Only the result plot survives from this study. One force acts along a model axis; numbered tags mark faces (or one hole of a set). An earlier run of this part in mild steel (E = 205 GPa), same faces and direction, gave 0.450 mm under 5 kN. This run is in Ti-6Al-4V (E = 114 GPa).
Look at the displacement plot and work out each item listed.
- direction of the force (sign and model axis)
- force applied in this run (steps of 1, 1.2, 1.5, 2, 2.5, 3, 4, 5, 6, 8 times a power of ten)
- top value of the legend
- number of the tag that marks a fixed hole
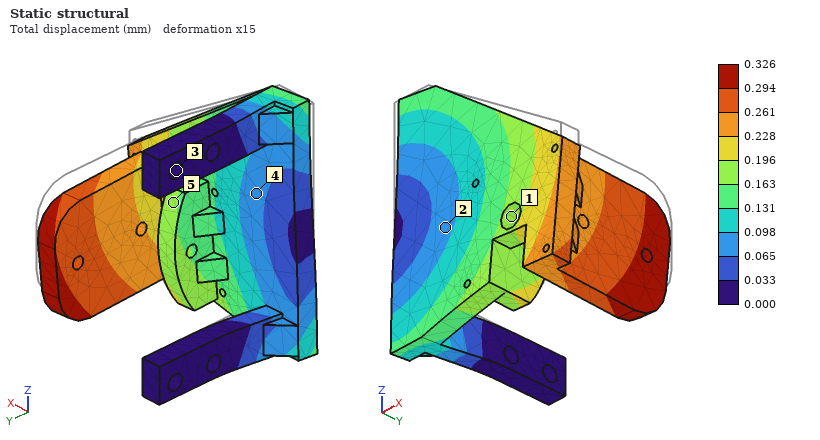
-Z
2 kN
0.326 mm
3
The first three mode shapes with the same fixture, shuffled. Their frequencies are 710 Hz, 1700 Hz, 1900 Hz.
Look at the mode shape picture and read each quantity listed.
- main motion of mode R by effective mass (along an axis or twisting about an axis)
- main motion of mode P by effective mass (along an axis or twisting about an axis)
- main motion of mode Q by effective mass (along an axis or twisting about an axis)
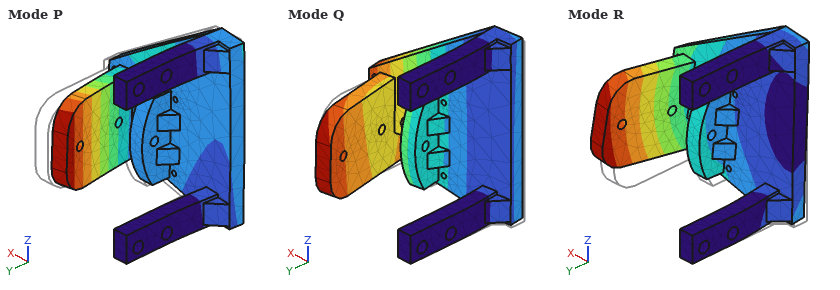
along Z
along X
along Y
